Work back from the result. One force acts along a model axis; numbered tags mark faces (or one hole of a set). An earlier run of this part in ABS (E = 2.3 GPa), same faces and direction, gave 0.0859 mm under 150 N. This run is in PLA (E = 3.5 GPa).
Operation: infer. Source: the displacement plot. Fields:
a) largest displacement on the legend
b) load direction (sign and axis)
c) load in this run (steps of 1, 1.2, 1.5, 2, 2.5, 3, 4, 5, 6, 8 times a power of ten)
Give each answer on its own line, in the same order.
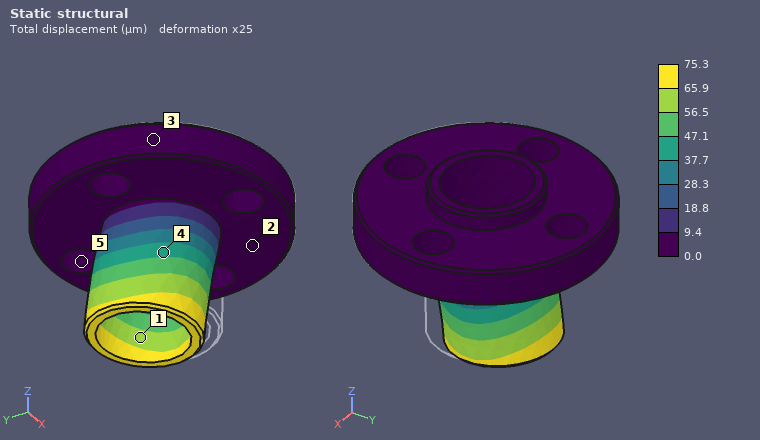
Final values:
75.3 µm
+Y
200 N
